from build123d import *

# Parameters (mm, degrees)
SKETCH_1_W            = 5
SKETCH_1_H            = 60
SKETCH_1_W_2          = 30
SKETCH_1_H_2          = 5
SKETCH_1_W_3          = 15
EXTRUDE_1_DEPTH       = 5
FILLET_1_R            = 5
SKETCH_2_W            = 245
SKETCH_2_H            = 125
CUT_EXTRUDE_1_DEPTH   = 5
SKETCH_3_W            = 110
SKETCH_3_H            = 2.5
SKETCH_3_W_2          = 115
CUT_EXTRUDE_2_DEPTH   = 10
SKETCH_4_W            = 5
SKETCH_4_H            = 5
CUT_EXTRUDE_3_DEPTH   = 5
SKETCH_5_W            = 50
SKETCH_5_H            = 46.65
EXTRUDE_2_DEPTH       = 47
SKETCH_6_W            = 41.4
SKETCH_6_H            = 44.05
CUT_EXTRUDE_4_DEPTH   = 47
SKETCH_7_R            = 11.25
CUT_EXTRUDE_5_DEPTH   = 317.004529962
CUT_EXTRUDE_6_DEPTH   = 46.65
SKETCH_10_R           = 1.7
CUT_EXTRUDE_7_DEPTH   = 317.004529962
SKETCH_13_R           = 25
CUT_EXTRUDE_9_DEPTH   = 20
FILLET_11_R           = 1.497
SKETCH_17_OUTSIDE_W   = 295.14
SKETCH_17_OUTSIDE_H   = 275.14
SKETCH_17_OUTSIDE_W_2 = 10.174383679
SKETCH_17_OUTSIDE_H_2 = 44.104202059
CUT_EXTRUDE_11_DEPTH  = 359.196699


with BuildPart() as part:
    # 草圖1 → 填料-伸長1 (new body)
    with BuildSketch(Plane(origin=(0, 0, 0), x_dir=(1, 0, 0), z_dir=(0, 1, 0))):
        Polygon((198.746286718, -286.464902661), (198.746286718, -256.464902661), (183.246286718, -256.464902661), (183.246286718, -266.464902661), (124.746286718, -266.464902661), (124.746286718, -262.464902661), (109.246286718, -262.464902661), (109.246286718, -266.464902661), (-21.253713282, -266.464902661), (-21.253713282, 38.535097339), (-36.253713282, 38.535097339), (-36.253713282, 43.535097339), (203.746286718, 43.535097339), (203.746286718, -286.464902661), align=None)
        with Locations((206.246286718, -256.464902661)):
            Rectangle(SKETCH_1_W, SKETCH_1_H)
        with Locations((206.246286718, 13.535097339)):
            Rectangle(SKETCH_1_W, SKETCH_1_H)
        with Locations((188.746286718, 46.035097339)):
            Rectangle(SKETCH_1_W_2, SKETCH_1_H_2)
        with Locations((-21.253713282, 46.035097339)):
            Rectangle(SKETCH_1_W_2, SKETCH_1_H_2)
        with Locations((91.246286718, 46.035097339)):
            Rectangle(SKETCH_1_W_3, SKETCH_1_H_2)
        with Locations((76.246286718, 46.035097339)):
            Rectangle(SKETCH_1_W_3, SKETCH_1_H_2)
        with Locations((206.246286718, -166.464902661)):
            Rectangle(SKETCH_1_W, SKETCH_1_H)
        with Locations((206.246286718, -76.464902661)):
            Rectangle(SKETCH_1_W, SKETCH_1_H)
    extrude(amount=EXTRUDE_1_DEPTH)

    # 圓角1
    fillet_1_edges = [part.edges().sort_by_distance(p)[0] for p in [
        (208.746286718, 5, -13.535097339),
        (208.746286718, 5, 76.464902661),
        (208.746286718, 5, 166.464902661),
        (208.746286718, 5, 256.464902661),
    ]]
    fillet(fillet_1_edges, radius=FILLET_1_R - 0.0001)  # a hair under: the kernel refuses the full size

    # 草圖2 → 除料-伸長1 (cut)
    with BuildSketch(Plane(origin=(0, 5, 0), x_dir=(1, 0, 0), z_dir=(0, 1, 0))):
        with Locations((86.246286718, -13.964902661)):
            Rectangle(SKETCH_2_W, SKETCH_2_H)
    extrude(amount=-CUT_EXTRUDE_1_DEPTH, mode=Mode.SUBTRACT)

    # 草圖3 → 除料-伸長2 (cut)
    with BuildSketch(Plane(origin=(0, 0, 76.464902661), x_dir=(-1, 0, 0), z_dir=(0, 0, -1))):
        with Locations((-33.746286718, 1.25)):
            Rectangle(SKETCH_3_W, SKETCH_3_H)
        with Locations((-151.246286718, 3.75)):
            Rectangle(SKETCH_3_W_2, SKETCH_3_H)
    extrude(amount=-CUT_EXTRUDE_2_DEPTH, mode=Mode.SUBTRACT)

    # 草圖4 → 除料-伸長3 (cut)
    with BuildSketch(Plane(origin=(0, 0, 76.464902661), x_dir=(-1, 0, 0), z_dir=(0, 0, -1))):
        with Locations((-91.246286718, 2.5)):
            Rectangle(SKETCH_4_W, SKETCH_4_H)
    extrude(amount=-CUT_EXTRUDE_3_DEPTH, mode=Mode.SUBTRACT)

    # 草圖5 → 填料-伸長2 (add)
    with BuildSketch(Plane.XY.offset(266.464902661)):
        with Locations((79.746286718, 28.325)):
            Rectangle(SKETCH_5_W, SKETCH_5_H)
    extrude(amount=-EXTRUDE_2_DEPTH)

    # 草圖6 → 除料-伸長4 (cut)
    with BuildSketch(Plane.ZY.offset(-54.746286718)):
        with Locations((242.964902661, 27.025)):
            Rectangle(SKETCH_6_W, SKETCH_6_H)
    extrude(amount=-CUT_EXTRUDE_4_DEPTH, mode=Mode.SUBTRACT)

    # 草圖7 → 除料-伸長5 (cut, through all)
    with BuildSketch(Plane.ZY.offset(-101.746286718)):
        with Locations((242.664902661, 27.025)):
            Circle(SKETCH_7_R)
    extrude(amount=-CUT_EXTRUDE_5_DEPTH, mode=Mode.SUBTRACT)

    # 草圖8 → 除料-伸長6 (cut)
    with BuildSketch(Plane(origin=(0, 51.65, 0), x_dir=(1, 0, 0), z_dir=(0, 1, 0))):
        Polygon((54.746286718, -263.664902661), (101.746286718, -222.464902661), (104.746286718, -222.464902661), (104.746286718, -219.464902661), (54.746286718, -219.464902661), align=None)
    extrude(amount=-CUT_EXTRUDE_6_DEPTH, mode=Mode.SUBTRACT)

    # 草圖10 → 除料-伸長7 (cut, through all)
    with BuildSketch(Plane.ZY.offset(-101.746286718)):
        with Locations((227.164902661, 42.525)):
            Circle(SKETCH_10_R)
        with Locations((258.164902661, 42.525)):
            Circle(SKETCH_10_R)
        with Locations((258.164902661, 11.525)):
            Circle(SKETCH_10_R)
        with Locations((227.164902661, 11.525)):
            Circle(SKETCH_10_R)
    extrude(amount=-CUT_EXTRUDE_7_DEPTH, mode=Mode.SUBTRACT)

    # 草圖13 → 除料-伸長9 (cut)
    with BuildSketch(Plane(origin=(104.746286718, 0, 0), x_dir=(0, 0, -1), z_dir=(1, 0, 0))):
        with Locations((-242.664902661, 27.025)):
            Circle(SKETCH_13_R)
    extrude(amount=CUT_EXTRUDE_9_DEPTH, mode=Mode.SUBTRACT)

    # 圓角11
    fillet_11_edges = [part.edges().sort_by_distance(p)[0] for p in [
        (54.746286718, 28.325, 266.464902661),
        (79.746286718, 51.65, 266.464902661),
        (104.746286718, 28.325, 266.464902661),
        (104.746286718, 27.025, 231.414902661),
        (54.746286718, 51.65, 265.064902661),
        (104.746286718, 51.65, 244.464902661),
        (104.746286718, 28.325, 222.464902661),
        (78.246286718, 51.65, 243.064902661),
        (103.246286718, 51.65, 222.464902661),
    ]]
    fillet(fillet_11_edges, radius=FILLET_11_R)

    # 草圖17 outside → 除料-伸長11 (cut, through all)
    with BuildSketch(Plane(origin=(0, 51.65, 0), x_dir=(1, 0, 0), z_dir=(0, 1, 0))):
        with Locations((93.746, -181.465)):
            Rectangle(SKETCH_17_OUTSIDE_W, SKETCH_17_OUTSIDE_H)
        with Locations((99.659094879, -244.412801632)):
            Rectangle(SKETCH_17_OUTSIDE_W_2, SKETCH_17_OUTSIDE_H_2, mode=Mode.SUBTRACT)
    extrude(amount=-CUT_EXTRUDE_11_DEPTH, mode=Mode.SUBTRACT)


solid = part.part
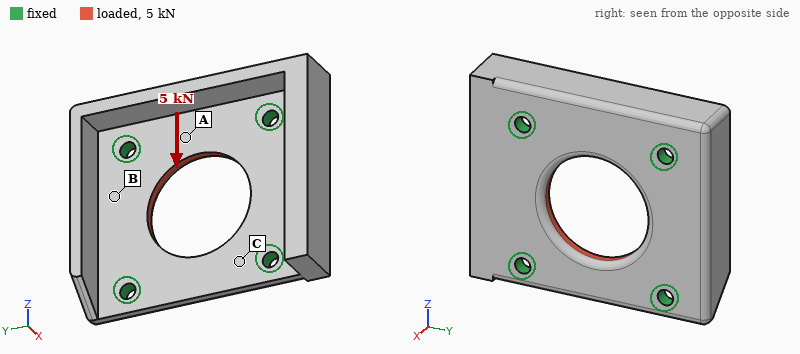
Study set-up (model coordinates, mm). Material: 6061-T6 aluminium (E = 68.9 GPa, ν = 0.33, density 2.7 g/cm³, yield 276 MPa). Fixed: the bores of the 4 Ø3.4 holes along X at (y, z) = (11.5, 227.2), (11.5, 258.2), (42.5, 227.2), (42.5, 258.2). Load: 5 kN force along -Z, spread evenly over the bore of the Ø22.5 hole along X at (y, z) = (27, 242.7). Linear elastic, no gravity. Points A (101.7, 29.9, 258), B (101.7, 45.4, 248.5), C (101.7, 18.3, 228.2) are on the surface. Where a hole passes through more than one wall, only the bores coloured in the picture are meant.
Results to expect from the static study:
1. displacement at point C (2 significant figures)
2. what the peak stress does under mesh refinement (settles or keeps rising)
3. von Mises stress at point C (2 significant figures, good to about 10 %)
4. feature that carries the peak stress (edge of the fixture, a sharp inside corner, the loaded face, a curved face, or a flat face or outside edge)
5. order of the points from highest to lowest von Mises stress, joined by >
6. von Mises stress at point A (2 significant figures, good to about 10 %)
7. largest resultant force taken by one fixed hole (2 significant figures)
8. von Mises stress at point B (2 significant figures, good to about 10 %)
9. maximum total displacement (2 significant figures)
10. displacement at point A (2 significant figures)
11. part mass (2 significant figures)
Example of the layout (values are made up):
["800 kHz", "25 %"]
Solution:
["9.1 µm", "keeps rising", "54 MPa", "edge of the fixture", "C > A > B", "35 MPa", "1.3 kN", "16 MPa", "21 µm", "11 µm", "23 g"]
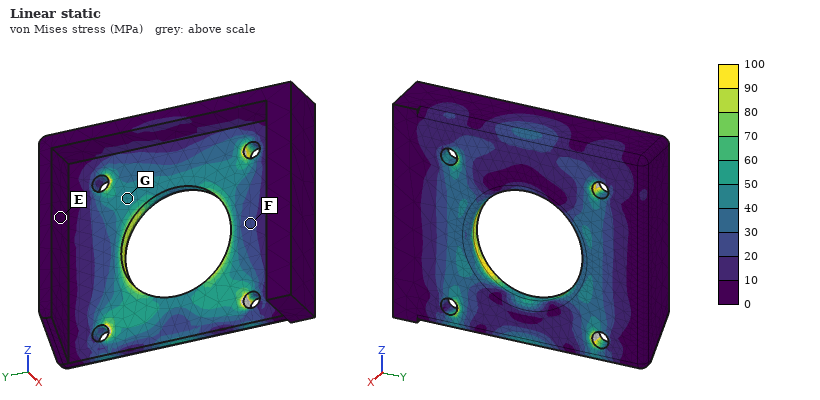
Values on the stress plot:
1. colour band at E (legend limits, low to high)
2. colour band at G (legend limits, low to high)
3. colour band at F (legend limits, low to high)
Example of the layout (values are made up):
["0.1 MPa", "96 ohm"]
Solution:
["0 to 10 MPa", "40 to 50 MPa", "20 to 30 MPa"]
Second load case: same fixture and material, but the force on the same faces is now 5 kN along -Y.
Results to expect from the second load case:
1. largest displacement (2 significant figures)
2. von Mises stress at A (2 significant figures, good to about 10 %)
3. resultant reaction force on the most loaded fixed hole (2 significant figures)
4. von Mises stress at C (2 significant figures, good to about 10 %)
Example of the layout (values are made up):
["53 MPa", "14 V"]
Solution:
["16 µm", "21 MPa", "1.3 kN", "31 MPa"]
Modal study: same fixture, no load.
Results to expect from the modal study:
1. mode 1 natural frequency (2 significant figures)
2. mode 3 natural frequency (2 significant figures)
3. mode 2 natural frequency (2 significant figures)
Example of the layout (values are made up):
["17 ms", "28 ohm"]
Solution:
["8900 Hz", "15 kHz", "13 kHz"]
